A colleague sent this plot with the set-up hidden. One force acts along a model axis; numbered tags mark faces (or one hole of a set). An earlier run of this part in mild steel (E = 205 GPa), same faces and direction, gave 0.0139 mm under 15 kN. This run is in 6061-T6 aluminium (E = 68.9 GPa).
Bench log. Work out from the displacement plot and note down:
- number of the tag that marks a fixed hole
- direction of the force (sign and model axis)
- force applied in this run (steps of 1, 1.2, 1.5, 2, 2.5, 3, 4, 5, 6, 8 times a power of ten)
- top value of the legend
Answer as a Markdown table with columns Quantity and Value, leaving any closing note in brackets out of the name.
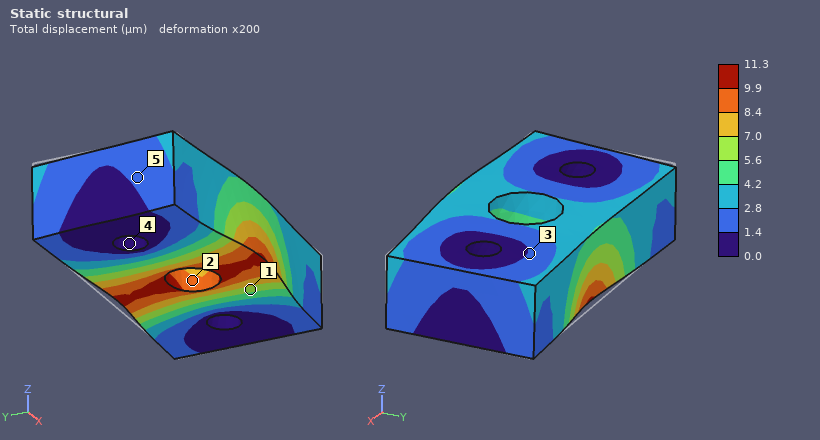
| Quantity | Value |
|---|---|
| number of the tag that marks a fixed hole | 4 |
| direction of the force | -Y |
| force applied in this run | 4 kN |
| top value of the legend | 11.3 µm |
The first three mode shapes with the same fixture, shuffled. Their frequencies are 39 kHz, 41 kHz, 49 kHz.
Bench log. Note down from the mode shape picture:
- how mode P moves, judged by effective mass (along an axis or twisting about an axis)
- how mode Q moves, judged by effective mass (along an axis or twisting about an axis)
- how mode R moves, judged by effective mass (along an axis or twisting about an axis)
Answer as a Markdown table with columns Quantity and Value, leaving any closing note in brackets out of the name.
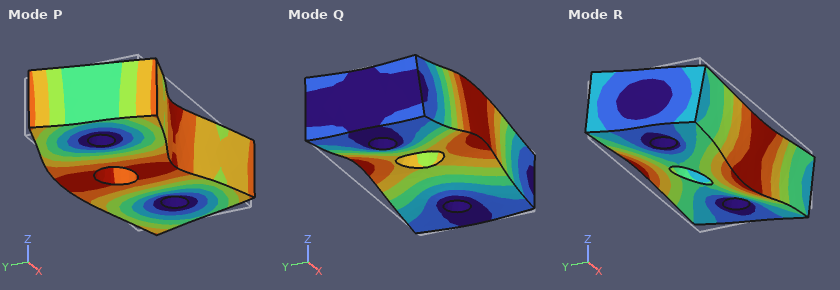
| Quantity | Value |
|---|---|
| how mode P moves, judged by effective mass | along Y |
| how mode Q moves, judged by effective mass | along Z |
| how mode R moves, judged by effective mass | twisting about X |
